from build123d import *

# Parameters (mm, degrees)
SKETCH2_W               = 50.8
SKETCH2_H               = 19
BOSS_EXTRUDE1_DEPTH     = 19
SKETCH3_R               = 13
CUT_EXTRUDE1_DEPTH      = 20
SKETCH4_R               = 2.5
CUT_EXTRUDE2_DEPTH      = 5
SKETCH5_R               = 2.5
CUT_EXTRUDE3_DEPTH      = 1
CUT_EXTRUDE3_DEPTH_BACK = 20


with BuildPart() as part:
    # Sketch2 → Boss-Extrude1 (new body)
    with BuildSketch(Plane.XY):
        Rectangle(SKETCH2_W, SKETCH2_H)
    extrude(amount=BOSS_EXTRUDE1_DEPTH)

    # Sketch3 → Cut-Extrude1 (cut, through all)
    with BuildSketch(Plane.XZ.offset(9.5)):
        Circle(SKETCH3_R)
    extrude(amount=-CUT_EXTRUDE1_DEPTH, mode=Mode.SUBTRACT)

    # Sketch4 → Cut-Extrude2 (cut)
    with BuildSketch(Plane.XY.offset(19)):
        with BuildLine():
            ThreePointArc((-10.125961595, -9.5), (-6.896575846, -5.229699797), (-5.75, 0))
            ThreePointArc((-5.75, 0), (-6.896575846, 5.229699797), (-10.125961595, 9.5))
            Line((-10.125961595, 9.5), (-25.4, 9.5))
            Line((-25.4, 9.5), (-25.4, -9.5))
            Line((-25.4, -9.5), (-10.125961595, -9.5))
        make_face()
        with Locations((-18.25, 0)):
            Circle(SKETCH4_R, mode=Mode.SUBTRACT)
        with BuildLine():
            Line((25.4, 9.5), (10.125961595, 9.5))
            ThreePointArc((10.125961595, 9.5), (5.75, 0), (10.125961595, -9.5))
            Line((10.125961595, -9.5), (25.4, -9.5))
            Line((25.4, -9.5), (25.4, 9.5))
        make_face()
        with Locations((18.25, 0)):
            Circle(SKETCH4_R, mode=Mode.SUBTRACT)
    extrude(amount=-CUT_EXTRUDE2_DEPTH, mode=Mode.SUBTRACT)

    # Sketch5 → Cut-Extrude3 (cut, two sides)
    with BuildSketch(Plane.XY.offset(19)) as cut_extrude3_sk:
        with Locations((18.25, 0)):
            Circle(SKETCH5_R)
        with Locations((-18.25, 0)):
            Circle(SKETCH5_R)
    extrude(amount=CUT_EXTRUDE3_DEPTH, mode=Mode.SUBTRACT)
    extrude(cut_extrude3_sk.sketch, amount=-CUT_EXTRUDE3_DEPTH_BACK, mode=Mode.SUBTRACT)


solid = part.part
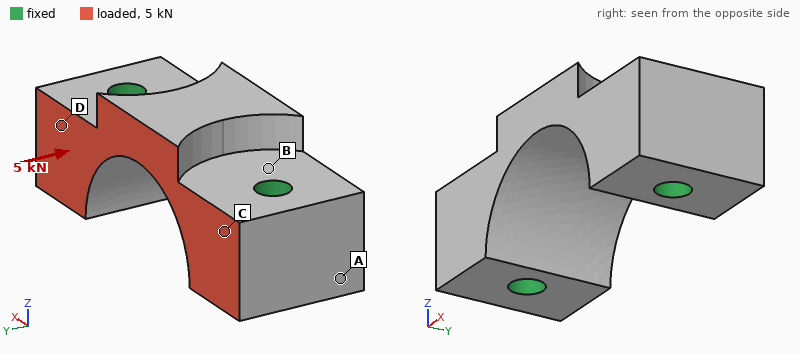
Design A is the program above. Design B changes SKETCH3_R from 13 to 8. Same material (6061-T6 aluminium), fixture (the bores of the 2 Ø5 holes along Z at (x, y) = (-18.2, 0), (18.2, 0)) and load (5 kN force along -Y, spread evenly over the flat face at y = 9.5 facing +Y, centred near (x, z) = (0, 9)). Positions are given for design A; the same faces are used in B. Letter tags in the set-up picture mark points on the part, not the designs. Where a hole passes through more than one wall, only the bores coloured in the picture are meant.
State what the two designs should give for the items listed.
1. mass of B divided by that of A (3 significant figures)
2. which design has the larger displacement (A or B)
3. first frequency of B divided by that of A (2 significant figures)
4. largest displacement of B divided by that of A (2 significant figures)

1.34
A
1.0
0.73
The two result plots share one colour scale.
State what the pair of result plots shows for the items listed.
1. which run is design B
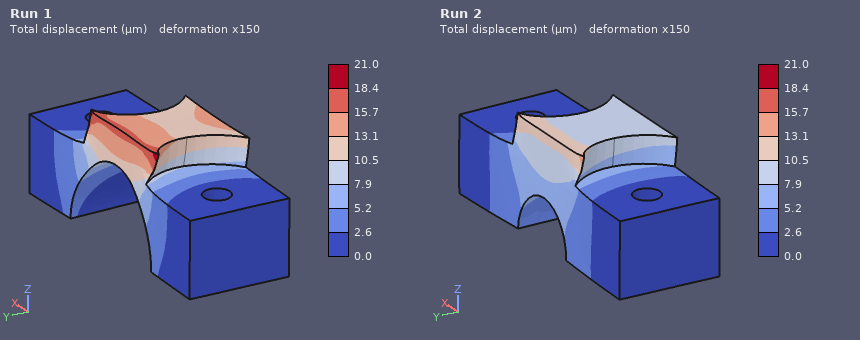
Run 2
